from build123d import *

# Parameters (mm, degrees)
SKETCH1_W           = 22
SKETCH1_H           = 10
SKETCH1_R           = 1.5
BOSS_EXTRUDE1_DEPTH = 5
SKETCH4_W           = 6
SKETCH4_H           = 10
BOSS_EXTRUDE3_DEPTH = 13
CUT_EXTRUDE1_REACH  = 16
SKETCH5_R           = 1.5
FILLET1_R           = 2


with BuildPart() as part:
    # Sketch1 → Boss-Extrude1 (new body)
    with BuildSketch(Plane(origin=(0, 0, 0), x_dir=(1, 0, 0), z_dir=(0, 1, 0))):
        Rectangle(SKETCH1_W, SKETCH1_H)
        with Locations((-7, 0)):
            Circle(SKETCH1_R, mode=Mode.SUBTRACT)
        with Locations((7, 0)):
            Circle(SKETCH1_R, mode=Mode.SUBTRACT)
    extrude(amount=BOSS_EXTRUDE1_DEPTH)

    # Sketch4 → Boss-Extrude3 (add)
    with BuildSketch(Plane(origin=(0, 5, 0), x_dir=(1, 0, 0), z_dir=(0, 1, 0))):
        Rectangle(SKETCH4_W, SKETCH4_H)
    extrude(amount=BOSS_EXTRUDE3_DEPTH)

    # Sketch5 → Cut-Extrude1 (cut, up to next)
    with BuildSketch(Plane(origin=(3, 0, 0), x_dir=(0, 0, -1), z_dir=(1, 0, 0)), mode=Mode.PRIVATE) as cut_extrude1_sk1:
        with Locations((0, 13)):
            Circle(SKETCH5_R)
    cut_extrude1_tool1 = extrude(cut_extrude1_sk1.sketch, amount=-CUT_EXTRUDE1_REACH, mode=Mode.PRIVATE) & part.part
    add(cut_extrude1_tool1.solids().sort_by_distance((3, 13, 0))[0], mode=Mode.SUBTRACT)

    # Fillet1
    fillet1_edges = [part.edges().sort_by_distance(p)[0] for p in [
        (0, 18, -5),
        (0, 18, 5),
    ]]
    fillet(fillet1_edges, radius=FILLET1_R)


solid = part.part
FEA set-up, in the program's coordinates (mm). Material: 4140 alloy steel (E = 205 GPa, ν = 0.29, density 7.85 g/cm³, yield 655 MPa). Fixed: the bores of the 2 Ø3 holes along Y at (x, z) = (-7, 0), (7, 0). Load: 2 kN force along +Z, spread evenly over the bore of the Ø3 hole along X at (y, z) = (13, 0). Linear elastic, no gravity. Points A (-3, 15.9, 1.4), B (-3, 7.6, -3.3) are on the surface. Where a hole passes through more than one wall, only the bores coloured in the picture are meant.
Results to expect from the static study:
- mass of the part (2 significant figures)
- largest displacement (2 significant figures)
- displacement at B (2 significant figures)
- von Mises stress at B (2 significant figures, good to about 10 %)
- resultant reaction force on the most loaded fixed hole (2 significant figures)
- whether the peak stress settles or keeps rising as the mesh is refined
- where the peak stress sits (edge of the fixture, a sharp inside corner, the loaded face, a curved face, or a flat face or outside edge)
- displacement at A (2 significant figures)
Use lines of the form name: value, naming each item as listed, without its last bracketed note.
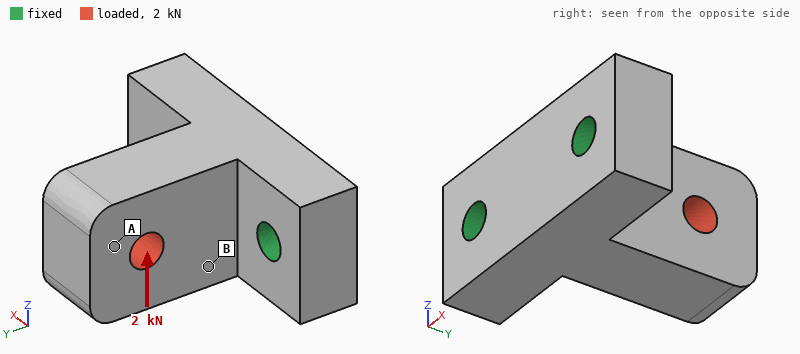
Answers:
mass of the part: 14 g
largest displacement: 47 µm
displacement at B: 16 µm
von Mises stress at B: 91 MPa
resultant reaction force on the most loaded fixed hole: 1.0 kN
whether the peak stress settles or keeps rising as the mesh is refined: keeps rising
where the peak stress sits: edge of the fixture
displacement at A: 40 µm
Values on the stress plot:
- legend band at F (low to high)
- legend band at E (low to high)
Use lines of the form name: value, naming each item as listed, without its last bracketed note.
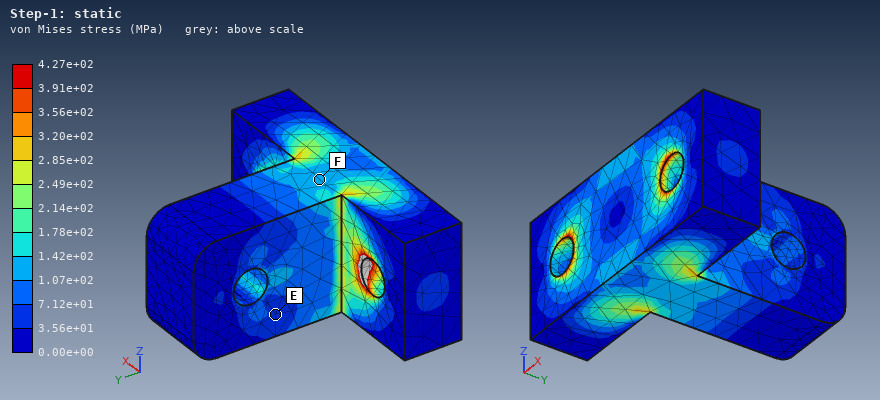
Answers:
legend band at F: 1.07e+02 to 1.42e+02 MPa
legend band at E: 3.56e+01 to 7.12e+01 MPa
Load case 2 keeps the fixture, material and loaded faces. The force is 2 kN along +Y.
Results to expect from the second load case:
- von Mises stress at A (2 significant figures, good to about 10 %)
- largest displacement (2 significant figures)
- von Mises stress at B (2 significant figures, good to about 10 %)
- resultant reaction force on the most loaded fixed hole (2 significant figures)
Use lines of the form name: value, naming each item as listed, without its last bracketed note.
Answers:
von Mises stress at A: 28 MPa
largest displacement: 4.2 µm
von Mises stress at B: 32 MPa
resultant reaction force on the most loaded fixed hole: 1.0 kN
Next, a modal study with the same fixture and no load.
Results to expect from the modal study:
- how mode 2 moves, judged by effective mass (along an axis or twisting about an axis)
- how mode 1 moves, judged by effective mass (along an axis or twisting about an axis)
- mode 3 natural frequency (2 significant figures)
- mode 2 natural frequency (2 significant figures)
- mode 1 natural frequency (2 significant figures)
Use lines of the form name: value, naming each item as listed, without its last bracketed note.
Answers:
how mode 2 moves, judged by effective mass: along X
how mode 1 moves, judged by effective mass: along Z
mode 3 natural frequency: 46 kHz
mode 2 natural frequency: 20 kHz
mode 1 natural frequency: 18 kHz
